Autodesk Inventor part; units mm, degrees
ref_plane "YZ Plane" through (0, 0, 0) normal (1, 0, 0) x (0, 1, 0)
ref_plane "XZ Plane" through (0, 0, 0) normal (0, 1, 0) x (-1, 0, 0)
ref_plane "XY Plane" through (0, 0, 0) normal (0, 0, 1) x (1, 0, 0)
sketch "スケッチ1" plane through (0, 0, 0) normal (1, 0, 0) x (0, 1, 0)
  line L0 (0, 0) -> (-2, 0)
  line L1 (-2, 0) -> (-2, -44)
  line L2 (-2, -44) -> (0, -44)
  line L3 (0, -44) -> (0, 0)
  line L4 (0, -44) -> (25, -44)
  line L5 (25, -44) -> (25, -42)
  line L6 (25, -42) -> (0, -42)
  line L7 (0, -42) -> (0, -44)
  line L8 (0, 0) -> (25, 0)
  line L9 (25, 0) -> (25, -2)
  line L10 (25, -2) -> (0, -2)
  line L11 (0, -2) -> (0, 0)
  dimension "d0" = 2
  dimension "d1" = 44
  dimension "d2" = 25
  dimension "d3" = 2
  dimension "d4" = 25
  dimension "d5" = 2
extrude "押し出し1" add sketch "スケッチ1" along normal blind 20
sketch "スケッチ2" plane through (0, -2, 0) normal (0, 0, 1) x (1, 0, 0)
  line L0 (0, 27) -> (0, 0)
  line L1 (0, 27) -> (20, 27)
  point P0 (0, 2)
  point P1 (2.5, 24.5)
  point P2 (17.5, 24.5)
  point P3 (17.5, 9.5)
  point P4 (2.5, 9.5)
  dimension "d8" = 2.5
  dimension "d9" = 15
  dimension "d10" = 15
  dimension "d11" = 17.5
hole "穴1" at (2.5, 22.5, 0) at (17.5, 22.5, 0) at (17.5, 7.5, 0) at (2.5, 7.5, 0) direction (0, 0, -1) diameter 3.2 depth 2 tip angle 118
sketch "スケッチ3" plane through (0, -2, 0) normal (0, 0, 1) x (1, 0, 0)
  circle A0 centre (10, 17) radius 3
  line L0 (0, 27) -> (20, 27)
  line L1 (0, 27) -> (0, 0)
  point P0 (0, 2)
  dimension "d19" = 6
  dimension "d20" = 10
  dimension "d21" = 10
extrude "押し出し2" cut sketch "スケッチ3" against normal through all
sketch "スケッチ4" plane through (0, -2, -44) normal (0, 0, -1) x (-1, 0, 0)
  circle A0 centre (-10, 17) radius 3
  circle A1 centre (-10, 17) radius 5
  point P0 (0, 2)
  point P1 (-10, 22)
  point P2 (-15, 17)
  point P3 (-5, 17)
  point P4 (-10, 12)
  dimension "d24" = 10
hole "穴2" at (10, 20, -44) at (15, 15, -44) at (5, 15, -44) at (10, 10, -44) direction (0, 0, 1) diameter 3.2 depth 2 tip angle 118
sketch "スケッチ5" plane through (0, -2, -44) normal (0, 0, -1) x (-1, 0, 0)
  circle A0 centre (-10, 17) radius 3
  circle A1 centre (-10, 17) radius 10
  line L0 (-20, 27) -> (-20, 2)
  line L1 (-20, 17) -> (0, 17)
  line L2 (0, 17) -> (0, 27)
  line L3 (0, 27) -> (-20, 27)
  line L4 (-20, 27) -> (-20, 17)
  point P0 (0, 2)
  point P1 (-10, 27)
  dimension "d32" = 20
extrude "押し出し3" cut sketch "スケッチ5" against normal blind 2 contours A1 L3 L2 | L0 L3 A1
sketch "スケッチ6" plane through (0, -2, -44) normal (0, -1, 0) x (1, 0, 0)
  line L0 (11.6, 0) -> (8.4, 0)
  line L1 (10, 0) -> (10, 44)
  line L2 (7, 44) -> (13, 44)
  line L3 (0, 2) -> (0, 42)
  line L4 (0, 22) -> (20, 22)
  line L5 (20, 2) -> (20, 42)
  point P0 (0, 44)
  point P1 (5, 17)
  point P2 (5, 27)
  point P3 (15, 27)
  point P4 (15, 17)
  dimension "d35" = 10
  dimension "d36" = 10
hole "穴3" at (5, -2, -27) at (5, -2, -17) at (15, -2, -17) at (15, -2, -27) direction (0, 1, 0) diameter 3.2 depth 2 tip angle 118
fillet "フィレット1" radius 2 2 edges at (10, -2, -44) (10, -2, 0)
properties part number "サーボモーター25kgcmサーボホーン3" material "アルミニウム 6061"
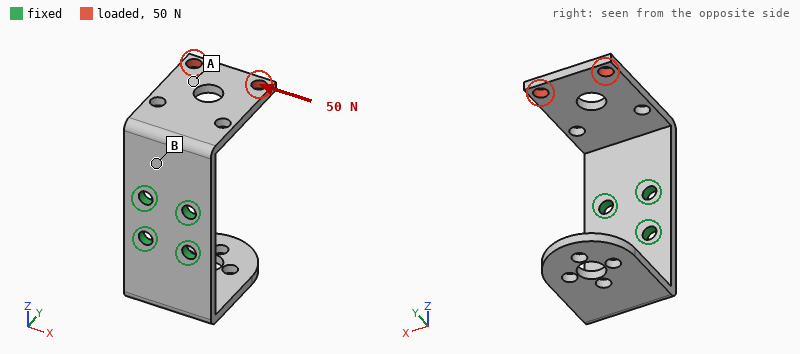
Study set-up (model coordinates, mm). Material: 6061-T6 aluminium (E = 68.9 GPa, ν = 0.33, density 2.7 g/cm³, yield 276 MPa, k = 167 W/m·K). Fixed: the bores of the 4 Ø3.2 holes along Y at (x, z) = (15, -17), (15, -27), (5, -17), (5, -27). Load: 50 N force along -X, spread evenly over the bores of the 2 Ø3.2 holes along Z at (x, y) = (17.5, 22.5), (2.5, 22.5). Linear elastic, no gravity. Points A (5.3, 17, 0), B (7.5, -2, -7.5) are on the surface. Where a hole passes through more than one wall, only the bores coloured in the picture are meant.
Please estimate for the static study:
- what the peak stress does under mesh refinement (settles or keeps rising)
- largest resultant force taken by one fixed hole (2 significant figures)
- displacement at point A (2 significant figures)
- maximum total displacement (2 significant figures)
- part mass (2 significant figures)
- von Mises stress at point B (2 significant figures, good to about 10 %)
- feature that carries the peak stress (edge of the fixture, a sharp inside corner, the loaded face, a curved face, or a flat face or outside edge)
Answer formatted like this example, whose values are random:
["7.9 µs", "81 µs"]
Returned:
["keeps rising", "110 N", "0.15 mm", "0.23 mm", "9.0 g", "55 MPa", "edge of the fixture"]
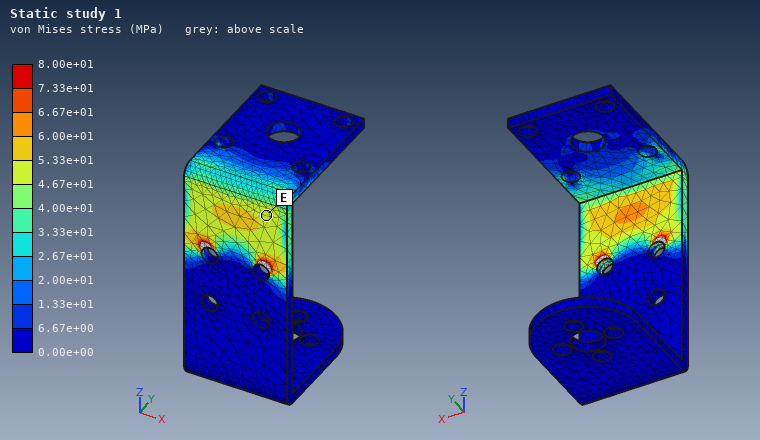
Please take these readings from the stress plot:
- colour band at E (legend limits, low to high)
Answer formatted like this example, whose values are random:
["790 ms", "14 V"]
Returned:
["4.67e+01 to 5.33e+01 MPa"]
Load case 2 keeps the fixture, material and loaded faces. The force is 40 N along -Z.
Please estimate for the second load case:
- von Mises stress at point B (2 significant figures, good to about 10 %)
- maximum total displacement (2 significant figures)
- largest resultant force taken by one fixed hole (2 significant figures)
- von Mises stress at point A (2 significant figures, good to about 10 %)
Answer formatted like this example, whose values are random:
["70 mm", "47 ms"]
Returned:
["61 MPa", "0.63 mm", "20 N", "21 MPa"]
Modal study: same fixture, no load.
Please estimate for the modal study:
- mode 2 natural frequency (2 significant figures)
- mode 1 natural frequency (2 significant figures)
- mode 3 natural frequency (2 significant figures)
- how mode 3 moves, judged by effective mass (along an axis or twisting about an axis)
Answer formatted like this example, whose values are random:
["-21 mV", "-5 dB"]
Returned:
["1500 Hz", "1300 Hz", "2400 Hz", "along X"]
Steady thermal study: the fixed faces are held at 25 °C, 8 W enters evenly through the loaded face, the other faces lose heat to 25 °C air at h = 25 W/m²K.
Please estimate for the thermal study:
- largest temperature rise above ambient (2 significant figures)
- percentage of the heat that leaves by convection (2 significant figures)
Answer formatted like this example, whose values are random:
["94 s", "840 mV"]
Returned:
["53 K", "13 %"]
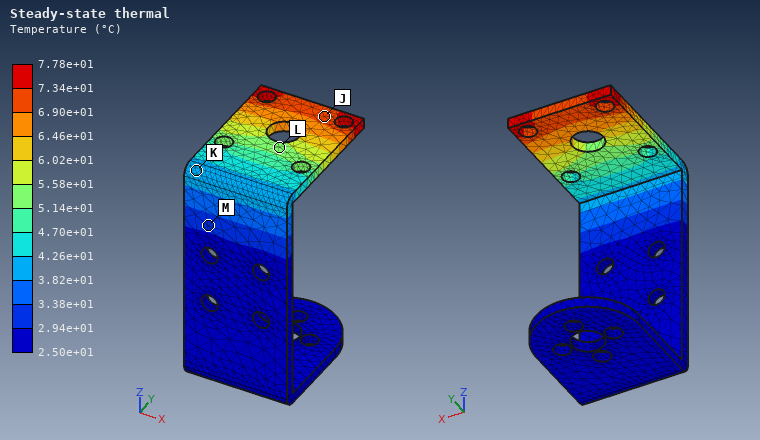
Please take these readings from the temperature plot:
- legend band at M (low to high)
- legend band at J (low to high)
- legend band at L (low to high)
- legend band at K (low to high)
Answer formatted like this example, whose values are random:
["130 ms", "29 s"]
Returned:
["2.94e+01 to 3.38e+01 °C", "6.90e+01 to 7.34e+01 °C", "5.14e+01 to 5.58e+01 °C", "3.82e+01 to 4.26e+01 °C"]
